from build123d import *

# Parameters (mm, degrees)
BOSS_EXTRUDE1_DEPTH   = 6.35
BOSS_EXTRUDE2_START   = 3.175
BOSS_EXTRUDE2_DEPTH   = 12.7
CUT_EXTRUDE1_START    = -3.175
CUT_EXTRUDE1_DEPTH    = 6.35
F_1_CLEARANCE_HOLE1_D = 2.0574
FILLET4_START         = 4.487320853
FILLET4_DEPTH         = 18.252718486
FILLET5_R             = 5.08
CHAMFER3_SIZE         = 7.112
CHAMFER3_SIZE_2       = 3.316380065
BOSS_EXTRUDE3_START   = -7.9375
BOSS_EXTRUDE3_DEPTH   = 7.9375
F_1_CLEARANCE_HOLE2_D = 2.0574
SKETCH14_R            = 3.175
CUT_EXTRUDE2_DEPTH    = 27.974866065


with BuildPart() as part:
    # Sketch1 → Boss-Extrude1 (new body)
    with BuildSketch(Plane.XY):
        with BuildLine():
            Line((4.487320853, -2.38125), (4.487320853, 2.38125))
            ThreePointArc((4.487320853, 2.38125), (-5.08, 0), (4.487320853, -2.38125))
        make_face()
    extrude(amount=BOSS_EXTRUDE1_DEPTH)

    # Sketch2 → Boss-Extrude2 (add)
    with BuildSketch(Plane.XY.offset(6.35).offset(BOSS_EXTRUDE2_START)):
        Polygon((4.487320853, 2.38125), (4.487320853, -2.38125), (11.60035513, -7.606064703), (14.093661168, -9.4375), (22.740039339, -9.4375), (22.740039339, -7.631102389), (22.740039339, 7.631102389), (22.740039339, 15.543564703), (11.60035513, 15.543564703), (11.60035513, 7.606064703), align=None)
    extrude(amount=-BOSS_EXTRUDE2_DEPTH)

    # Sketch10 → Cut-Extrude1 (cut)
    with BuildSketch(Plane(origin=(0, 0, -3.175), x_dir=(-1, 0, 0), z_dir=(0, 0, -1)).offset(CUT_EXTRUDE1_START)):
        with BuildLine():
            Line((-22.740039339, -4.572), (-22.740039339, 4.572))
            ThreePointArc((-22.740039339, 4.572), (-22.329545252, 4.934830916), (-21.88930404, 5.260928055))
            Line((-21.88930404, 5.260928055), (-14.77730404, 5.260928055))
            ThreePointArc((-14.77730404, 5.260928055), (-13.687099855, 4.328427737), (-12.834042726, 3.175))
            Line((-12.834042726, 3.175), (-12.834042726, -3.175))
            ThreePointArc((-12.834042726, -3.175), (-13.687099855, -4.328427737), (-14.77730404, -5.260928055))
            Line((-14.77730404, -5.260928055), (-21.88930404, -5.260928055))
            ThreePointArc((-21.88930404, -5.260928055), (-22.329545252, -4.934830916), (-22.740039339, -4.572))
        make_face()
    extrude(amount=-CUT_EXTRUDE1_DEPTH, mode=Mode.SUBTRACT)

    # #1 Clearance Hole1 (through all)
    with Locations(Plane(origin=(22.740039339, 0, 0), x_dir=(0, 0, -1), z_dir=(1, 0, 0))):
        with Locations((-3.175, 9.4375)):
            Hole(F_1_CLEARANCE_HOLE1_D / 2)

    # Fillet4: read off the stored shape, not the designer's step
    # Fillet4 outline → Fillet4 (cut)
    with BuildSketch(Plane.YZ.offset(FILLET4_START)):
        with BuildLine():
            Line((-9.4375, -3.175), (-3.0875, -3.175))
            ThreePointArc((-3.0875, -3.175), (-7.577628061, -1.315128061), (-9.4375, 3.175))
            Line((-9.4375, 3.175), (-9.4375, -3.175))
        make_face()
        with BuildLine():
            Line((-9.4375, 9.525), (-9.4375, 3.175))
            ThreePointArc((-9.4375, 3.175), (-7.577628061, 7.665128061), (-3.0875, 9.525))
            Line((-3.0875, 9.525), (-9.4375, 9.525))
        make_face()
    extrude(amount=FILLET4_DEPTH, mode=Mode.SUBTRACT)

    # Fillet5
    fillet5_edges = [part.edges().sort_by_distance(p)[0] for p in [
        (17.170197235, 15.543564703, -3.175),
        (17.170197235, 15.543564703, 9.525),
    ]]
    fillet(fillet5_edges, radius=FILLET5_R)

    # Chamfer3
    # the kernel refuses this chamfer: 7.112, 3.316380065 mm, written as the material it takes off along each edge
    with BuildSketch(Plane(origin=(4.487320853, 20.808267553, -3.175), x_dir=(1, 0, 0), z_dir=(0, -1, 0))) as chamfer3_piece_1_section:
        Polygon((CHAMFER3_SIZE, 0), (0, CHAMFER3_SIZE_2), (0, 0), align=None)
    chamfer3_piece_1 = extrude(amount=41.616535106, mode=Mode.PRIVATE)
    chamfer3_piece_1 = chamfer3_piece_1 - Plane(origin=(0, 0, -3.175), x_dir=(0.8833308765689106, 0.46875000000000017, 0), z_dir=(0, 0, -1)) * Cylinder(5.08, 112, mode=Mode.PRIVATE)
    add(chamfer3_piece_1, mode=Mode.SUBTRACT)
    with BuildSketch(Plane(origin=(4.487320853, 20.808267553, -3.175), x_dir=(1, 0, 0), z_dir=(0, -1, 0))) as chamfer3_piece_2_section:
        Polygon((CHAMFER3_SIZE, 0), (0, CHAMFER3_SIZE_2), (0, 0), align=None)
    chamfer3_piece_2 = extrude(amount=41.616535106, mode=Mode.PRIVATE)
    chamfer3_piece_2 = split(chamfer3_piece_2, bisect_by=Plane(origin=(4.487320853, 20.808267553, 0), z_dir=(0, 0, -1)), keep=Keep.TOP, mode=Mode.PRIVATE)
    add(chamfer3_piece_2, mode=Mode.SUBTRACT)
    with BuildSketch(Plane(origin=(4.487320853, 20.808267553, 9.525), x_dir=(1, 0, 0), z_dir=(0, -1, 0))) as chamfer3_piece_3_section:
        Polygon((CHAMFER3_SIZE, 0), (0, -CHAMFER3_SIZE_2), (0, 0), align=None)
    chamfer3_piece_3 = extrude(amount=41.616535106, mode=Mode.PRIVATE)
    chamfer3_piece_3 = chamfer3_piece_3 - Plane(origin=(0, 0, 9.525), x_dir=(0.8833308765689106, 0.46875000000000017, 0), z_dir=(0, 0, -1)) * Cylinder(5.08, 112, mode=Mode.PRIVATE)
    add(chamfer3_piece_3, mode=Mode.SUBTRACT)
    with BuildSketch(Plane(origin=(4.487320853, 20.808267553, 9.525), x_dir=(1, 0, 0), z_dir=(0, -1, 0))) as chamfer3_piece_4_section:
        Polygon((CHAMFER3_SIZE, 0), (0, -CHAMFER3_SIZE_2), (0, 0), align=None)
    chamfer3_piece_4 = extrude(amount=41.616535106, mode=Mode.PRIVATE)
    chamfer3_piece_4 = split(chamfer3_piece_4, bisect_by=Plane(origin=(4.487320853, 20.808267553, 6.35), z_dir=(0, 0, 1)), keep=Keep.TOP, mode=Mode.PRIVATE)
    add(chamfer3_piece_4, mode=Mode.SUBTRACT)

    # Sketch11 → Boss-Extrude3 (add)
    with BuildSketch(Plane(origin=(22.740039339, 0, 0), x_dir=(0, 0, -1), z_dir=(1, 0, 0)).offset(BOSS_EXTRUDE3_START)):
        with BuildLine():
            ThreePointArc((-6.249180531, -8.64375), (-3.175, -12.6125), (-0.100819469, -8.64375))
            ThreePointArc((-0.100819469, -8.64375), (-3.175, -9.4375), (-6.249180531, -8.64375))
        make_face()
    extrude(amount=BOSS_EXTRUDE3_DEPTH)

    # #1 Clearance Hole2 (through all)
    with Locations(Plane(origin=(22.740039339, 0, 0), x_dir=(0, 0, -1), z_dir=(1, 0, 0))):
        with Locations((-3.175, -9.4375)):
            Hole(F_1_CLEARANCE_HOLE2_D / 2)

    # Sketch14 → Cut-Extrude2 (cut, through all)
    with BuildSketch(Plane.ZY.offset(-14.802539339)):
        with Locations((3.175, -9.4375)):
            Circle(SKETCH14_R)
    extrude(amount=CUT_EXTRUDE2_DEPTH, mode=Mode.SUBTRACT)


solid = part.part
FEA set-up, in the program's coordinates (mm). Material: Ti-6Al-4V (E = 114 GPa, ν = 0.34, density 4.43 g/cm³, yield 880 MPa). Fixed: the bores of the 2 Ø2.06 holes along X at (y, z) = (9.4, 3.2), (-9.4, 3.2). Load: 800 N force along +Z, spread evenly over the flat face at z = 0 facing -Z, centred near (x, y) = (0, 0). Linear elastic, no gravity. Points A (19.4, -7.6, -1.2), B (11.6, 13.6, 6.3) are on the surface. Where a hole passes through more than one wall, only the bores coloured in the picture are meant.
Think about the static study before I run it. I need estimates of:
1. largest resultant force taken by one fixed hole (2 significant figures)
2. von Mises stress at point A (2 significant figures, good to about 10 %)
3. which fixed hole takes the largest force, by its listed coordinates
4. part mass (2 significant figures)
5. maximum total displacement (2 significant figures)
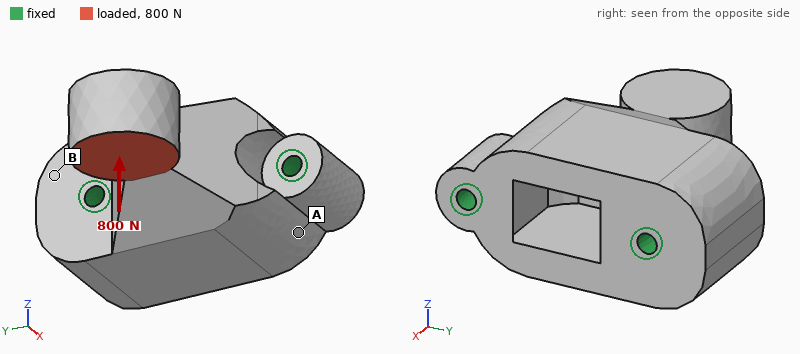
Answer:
500 N
43 MPa
(9.4, 3.2)
17 g
43 µm
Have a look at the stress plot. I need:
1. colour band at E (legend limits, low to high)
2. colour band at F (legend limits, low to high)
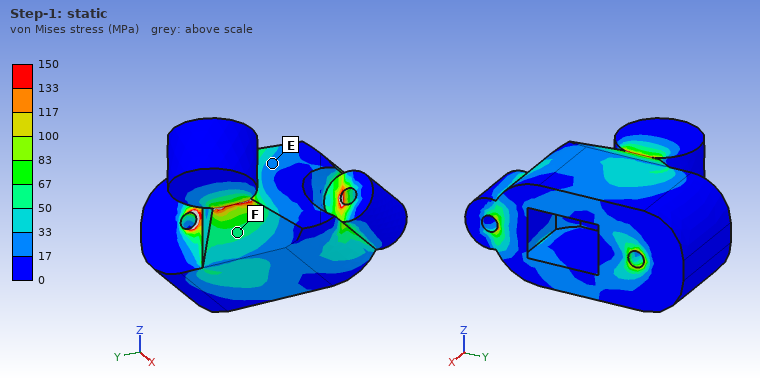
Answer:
17 to 33 MPa
50 to 67 MPa
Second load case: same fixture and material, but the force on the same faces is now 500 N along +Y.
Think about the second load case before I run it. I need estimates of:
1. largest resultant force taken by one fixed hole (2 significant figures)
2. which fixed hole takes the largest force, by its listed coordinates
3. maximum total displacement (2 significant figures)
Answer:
580 N
(9.4, 3.2)
22 µm
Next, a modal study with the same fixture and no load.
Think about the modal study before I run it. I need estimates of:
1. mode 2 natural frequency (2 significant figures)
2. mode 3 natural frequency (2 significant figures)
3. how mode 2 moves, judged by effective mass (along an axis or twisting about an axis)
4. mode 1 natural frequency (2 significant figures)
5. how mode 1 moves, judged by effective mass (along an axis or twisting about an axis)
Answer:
20 kHz
41 kHz
along Y
15 kHz
along Z
